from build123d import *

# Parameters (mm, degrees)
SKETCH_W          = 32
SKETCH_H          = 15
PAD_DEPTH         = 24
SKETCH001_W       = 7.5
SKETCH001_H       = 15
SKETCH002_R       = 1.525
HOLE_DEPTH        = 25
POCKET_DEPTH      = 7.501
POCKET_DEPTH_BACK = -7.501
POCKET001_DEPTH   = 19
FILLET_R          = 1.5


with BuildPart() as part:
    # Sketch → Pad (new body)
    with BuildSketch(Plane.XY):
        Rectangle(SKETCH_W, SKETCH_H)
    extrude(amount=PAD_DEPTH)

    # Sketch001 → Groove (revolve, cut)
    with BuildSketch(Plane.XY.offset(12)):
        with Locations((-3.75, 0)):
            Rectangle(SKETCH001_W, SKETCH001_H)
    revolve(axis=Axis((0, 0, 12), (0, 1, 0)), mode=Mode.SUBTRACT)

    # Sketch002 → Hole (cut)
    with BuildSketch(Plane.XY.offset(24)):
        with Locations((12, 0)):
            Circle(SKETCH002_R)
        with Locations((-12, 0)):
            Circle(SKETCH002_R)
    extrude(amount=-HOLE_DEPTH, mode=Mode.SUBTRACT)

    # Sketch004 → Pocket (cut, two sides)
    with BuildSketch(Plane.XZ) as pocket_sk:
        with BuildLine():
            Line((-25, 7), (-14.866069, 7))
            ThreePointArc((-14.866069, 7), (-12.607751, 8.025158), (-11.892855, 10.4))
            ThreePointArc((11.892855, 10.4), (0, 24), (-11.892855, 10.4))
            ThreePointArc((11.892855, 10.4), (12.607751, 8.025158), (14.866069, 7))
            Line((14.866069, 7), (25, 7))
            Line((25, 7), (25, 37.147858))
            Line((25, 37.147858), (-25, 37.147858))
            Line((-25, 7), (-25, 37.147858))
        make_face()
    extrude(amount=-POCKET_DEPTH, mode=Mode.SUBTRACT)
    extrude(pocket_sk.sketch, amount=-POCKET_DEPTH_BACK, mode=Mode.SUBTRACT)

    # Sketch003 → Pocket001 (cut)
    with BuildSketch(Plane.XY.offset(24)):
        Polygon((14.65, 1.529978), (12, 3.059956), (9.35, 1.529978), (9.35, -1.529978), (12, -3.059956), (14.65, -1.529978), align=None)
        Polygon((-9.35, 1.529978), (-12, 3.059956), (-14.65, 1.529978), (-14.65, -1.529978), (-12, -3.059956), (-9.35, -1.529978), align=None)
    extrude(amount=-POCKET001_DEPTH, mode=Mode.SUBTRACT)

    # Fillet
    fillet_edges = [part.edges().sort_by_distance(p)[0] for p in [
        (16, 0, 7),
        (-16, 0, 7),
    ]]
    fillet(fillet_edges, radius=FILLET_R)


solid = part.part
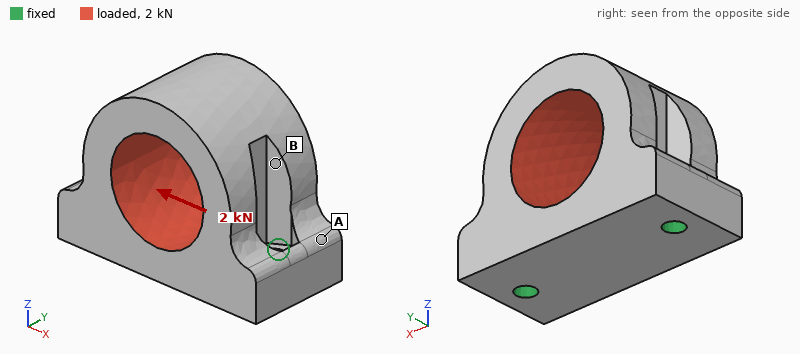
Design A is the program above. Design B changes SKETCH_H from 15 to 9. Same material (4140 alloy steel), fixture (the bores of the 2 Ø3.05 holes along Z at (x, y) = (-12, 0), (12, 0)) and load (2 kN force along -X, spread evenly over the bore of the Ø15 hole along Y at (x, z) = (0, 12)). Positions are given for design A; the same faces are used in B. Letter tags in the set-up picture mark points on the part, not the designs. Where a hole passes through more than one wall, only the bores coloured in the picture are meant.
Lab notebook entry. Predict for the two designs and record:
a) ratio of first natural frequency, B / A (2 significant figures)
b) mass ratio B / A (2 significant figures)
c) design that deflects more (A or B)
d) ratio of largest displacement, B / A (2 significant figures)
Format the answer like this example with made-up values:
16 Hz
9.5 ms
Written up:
1.0
0.57
B
1.8
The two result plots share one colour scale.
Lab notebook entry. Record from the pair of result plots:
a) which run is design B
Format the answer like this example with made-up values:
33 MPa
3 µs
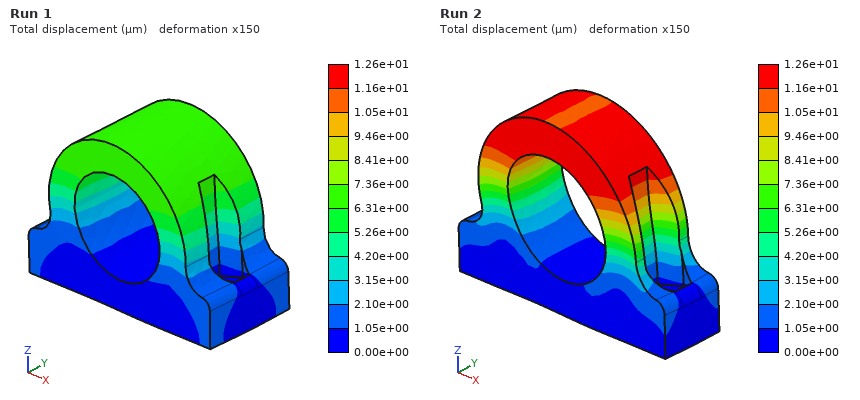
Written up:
Run 2
